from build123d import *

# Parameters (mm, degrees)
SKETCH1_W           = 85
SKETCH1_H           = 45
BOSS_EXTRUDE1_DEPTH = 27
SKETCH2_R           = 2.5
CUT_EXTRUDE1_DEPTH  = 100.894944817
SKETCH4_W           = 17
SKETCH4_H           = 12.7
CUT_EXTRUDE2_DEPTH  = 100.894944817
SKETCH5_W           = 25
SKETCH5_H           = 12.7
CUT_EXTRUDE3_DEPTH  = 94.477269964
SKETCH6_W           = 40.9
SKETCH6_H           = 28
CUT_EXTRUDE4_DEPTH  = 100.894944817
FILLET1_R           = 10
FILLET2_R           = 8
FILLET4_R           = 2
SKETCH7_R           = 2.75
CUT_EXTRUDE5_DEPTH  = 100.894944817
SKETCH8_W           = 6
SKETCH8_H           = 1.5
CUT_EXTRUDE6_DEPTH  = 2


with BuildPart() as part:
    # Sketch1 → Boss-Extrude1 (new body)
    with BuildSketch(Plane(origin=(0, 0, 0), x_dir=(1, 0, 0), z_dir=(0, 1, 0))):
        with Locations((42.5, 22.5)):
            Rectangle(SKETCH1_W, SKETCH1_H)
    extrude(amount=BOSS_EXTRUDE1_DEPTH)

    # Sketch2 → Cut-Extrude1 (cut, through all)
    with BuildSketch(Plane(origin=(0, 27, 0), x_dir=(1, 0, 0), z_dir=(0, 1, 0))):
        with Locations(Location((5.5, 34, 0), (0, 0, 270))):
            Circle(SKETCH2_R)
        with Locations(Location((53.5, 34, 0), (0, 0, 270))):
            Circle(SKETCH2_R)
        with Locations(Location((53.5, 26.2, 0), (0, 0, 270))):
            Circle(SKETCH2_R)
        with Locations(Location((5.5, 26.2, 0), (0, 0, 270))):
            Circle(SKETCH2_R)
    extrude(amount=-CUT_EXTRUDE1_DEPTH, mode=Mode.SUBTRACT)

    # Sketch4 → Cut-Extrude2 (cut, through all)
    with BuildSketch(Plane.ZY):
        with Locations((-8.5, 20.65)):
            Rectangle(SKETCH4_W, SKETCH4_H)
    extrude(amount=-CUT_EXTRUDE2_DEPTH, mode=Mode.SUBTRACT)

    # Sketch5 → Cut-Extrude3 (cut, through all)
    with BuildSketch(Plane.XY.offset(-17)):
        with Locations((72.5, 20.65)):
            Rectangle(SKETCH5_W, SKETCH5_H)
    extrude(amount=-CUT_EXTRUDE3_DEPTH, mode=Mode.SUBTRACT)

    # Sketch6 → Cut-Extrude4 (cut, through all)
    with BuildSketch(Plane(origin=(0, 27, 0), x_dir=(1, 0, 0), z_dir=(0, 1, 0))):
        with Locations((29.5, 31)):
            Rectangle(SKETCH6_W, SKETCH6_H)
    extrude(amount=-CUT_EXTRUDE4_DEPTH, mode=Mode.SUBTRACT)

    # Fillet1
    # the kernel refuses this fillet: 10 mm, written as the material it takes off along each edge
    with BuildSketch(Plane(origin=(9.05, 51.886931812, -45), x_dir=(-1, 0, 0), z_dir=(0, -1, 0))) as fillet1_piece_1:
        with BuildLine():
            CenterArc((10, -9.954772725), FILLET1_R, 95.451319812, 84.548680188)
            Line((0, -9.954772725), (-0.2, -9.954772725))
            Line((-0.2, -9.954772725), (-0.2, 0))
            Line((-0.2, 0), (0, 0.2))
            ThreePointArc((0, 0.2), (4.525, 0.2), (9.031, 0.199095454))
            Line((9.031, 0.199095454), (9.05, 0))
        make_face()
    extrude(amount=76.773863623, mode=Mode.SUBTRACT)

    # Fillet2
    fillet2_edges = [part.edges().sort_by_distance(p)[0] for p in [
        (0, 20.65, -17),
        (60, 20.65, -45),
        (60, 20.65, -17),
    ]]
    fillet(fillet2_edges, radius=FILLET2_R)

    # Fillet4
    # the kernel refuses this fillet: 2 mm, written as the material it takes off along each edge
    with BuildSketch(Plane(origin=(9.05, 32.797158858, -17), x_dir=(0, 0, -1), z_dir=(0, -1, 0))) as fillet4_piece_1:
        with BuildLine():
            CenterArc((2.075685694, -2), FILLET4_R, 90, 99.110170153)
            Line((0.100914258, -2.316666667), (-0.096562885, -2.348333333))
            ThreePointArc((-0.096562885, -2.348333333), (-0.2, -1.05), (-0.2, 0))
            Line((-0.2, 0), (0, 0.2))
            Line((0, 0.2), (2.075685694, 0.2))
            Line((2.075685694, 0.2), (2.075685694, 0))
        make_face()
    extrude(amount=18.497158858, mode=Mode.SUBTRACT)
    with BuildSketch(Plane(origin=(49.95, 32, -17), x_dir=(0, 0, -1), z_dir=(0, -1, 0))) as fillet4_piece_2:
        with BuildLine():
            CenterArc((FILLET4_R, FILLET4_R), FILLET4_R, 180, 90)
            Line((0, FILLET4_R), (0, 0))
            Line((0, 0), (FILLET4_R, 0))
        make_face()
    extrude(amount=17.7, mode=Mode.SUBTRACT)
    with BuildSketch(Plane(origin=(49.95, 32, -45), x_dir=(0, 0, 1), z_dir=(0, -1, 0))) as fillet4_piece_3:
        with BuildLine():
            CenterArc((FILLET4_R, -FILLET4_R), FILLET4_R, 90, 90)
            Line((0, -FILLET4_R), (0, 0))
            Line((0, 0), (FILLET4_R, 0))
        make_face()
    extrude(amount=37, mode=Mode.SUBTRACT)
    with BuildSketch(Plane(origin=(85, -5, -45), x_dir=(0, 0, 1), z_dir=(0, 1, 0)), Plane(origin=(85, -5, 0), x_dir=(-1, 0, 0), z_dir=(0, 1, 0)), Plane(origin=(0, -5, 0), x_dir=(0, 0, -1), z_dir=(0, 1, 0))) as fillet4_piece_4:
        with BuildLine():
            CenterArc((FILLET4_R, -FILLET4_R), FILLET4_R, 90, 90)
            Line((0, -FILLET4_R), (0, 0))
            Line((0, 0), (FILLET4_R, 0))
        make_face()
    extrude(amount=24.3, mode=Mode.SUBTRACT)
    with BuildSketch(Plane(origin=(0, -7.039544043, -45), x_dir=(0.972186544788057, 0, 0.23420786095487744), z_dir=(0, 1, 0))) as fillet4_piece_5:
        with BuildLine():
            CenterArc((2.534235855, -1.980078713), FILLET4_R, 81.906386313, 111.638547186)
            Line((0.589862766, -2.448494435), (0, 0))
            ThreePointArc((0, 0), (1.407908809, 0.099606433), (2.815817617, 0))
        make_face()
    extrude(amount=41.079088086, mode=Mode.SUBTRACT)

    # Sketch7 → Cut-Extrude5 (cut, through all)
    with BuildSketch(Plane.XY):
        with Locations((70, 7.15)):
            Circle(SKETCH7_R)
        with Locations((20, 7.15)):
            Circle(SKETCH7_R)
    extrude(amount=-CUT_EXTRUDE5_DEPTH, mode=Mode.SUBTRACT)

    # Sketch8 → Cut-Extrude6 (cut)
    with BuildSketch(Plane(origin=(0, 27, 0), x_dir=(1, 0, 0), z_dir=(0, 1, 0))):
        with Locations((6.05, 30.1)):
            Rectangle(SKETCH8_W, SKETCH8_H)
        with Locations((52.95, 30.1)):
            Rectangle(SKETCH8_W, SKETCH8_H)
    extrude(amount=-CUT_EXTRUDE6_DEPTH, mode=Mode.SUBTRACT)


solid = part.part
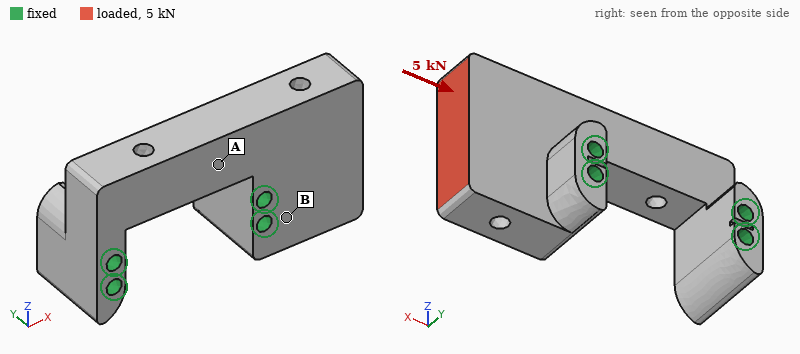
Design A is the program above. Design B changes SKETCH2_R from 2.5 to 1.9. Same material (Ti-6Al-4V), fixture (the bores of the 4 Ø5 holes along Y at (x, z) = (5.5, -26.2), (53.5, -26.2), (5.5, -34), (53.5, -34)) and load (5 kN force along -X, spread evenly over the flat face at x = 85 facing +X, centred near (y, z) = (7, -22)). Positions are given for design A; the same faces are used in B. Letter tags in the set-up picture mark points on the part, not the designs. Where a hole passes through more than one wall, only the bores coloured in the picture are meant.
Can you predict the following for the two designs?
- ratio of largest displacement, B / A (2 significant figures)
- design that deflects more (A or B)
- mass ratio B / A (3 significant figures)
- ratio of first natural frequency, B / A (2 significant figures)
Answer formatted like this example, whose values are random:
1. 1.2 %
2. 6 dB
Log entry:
1. 1.1
2. B
3. 1.02
4. 0.97
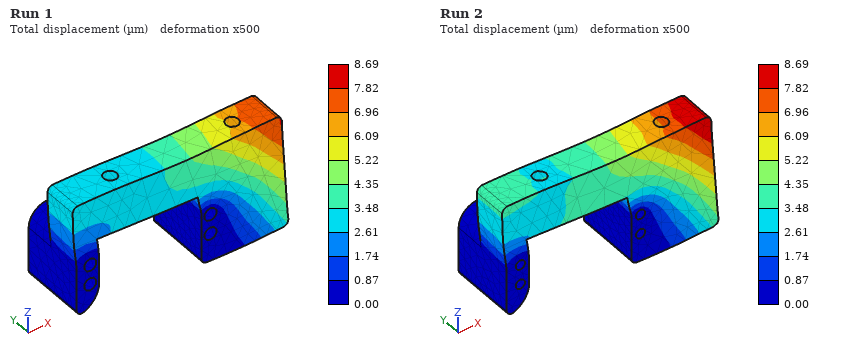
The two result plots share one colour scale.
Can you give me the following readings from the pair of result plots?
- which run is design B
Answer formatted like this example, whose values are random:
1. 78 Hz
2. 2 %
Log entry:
1. Run 2
